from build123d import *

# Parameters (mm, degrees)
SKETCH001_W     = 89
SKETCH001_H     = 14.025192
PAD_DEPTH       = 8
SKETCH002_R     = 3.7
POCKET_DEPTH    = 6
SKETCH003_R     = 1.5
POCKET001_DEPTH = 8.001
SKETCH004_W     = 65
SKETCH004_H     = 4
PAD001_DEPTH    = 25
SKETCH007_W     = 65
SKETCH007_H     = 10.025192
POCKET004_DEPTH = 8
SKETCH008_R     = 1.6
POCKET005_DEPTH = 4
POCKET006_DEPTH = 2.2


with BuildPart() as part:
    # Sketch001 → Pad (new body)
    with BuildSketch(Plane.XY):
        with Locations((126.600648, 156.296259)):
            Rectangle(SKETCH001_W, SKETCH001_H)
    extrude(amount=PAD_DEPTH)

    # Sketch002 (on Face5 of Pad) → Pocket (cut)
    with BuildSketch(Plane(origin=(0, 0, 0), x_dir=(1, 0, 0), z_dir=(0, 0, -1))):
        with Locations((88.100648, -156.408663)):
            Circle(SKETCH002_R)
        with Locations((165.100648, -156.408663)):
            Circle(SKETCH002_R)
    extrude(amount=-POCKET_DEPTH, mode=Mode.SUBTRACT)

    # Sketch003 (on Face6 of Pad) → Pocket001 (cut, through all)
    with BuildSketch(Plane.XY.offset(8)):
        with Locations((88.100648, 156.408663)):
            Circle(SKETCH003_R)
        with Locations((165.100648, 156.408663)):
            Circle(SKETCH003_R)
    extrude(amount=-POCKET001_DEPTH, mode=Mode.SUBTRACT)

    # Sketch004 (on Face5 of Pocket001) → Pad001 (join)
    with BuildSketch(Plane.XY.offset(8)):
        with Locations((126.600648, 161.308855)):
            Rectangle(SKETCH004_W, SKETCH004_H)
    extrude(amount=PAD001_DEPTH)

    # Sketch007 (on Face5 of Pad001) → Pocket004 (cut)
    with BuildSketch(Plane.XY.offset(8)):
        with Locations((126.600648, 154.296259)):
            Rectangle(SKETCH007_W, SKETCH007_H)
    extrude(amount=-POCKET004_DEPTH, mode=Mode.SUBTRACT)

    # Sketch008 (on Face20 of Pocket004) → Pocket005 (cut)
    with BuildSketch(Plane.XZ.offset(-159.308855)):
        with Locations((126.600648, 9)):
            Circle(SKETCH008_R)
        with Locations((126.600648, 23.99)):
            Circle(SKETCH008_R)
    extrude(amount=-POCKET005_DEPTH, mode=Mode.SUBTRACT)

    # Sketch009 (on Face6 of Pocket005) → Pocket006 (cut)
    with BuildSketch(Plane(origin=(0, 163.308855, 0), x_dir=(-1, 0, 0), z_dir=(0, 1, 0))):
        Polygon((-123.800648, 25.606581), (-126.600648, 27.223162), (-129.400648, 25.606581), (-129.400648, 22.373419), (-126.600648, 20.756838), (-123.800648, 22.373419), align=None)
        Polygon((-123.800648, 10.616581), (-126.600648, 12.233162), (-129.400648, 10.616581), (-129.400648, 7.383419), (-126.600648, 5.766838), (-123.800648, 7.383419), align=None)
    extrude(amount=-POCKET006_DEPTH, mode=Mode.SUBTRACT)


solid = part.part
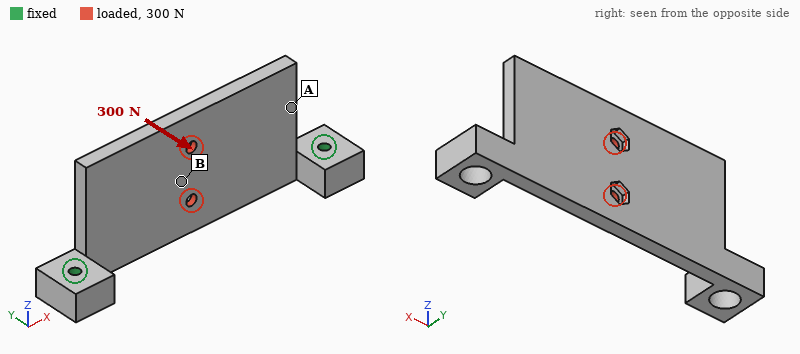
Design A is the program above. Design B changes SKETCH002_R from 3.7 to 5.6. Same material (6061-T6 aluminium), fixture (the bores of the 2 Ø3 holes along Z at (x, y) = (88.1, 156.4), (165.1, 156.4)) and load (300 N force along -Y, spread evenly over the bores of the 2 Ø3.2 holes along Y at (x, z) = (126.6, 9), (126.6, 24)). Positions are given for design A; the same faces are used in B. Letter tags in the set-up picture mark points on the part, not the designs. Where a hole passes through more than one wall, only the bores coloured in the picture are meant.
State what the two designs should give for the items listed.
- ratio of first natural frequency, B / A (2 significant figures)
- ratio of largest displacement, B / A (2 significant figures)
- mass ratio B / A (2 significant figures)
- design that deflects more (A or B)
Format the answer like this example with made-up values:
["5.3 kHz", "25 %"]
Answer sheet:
["0.90", "1.2", "0.94", "B"]
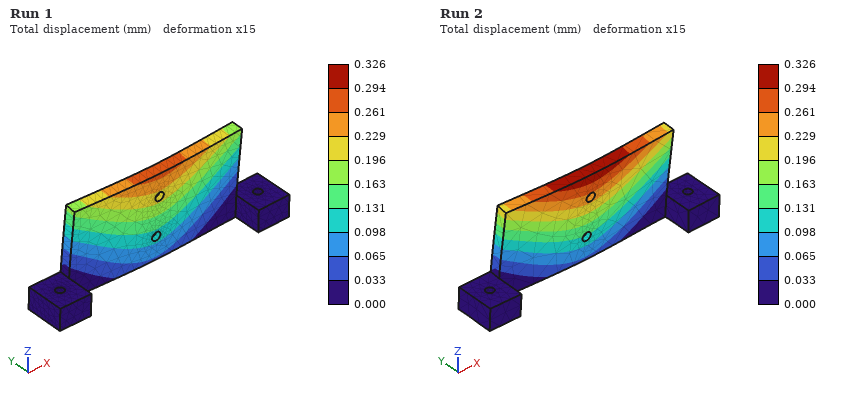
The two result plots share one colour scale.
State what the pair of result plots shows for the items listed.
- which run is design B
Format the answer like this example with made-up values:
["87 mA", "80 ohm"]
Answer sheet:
["Run 2"]
